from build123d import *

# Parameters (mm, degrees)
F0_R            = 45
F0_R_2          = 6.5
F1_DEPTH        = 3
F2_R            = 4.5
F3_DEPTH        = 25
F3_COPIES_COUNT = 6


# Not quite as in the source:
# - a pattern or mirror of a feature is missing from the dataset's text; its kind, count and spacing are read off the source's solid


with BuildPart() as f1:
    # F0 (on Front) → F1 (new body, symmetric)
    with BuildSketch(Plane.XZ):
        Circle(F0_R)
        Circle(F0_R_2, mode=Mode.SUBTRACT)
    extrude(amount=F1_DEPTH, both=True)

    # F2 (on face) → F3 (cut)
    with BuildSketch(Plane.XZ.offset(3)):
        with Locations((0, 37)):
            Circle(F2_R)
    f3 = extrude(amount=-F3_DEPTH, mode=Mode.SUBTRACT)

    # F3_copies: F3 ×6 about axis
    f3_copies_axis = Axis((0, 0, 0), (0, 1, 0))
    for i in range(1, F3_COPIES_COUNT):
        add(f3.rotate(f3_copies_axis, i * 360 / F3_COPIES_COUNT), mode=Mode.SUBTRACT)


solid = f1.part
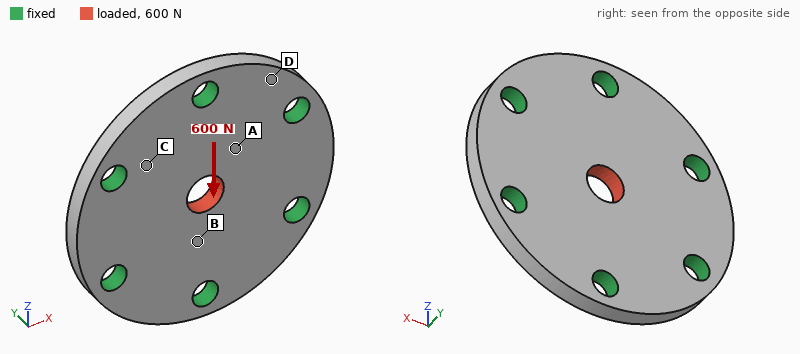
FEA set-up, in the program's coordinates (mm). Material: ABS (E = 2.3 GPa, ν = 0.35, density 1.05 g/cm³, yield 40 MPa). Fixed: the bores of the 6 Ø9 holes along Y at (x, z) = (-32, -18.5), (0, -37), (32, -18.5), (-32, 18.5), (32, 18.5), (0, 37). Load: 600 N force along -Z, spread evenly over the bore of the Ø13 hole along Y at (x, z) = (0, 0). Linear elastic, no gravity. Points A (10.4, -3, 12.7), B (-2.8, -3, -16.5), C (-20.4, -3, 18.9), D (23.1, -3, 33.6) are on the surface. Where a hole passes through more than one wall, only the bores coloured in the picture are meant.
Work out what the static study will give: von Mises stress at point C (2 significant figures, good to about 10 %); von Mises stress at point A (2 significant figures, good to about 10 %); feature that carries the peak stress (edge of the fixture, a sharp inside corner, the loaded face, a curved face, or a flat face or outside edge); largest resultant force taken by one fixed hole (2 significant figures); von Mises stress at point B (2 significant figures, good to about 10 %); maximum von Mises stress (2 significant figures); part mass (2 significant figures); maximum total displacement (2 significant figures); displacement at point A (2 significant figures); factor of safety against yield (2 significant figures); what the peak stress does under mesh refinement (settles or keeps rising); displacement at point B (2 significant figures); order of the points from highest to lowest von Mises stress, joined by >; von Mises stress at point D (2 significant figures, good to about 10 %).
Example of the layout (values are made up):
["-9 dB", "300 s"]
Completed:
["0.67 MPa", "1.2 MPa", "the loaded face", "160 N", "1.7 MPa", "4.2 MPa", "37 g", "21 µm", "11 µm", "9.4", "settles", "12 µm", "B > A > C > D", "0.34 MPa"]
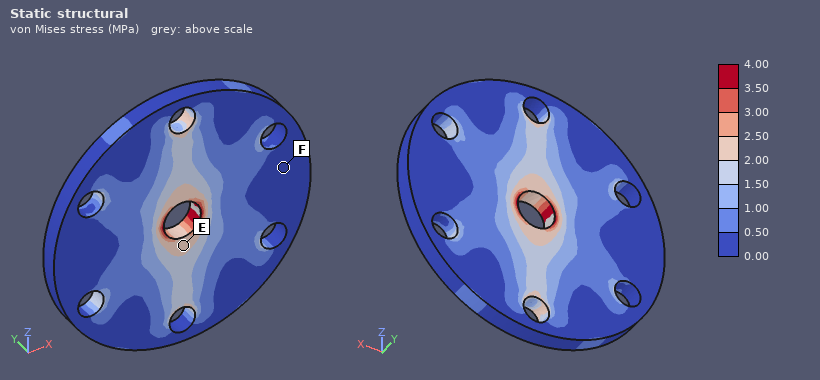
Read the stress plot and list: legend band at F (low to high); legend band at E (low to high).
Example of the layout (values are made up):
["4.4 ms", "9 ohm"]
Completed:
["0.00 to 0.50 MPa", "2.00 to 2.50 MPa"]
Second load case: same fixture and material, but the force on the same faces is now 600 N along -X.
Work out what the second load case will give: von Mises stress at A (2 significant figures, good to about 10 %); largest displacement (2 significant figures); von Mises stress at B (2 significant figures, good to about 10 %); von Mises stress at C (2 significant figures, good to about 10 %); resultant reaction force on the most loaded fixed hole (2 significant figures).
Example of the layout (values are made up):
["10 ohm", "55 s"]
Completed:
["1.2 MPa", "21 µm", "0.59 MPa", "0.98 MPa", "140 N"]
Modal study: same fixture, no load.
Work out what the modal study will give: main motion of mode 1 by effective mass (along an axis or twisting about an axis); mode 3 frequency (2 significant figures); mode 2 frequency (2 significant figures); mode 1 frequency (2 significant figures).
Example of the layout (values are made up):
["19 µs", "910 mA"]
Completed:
["along Y", "5700 Hz", "5700 Hz", "3100 Hz"]
